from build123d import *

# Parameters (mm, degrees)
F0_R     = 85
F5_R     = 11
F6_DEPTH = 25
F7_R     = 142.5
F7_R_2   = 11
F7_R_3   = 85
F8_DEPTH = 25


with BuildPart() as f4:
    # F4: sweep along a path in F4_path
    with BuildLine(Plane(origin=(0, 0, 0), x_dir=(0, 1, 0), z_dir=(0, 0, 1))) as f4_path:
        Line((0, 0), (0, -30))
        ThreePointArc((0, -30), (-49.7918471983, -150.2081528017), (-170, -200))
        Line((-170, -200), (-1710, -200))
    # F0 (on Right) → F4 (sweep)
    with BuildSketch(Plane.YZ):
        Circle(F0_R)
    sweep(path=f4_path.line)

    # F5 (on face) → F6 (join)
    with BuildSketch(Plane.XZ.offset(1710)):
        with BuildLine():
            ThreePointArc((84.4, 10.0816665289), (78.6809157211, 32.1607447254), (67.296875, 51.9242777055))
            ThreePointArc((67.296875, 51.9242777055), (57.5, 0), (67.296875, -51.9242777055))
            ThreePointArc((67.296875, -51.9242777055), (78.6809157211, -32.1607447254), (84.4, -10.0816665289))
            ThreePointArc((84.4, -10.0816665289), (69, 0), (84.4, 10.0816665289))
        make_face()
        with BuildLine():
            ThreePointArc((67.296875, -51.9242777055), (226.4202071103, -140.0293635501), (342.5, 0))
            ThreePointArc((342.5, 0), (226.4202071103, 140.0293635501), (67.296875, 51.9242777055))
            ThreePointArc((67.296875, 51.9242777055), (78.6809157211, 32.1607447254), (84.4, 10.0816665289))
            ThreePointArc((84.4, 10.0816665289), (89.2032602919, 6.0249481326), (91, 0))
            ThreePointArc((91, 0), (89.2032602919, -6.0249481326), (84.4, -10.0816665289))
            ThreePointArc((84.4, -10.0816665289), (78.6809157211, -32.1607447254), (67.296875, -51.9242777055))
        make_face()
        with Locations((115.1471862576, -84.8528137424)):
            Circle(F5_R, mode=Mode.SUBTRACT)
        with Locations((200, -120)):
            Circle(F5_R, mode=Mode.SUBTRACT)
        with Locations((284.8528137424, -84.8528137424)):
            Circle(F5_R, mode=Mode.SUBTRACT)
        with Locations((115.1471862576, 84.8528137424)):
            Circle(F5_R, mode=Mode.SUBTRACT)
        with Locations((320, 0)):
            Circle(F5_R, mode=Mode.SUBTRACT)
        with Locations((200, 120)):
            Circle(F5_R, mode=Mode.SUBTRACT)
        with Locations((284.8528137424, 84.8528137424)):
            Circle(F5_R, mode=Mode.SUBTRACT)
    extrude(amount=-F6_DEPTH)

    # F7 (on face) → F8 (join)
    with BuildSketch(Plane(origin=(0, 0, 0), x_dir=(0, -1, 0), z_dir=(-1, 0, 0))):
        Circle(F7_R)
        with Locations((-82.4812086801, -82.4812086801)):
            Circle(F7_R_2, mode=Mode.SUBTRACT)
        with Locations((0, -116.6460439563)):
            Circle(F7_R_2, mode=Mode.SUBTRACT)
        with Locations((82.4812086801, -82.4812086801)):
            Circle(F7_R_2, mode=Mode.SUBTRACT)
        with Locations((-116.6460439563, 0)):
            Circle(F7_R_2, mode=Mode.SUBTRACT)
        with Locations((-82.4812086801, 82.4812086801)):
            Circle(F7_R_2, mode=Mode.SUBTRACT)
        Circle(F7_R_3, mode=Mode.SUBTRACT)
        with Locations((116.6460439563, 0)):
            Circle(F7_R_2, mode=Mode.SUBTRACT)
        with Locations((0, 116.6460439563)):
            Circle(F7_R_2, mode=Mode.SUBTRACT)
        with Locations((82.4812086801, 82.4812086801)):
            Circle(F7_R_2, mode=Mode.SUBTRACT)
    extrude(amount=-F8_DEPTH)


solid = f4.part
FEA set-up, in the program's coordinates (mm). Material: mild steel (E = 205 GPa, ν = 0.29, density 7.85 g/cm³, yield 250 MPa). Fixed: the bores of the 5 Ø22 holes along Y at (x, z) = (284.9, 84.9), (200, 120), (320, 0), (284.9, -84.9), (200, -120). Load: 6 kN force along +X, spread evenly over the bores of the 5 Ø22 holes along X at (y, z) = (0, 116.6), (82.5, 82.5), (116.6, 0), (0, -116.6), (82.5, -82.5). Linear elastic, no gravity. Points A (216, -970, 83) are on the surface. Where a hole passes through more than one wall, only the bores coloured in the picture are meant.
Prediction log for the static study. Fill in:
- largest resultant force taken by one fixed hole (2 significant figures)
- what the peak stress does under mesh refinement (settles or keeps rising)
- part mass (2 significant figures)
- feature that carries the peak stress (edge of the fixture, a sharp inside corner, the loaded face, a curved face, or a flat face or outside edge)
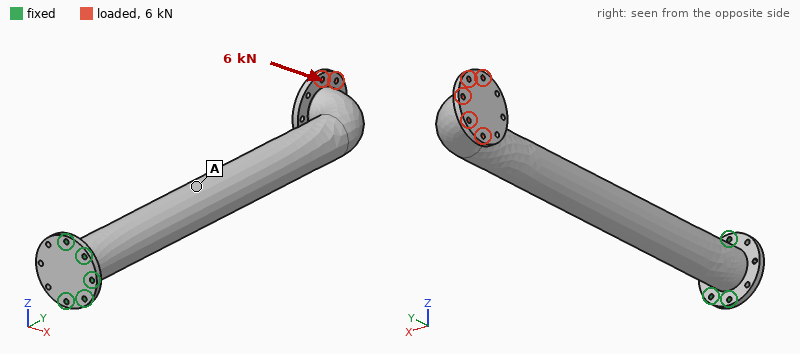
53 kN
keeps rising
340 kg
edge of the fixture
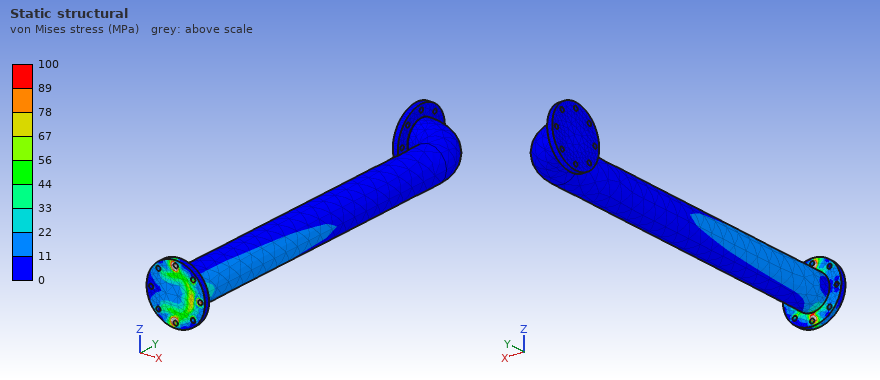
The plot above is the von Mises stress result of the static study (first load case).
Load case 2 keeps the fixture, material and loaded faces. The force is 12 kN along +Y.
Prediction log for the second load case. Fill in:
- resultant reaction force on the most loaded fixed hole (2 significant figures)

17 kN
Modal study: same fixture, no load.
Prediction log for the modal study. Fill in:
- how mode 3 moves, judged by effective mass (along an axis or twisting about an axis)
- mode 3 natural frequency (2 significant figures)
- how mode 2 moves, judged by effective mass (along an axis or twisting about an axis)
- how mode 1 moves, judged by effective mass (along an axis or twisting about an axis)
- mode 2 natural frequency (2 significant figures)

along X
170 Hz
along Z
along X
30 Hz
